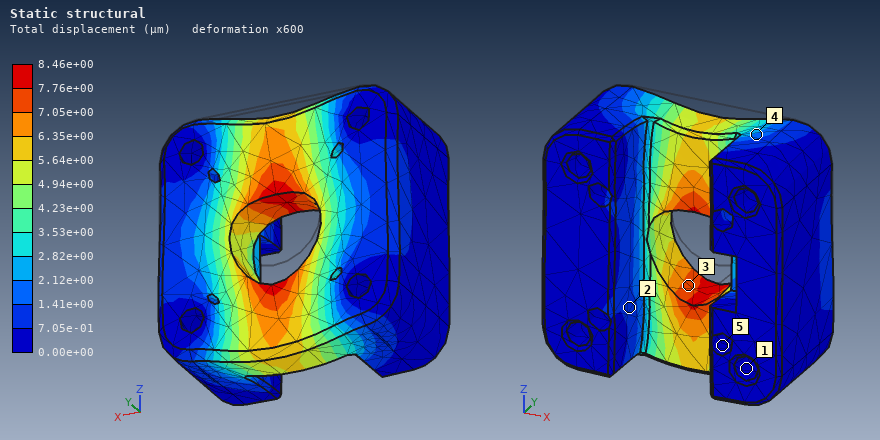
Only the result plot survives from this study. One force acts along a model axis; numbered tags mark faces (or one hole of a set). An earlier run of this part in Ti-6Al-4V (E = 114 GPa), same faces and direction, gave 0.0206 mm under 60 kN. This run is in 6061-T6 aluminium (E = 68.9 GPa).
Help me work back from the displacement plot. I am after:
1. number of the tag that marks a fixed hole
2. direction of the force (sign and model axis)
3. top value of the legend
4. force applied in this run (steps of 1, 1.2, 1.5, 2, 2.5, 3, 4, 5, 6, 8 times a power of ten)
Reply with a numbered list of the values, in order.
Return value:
1. 1
2. -Z
3. 8.46e+00 µm
4. 15 kN
